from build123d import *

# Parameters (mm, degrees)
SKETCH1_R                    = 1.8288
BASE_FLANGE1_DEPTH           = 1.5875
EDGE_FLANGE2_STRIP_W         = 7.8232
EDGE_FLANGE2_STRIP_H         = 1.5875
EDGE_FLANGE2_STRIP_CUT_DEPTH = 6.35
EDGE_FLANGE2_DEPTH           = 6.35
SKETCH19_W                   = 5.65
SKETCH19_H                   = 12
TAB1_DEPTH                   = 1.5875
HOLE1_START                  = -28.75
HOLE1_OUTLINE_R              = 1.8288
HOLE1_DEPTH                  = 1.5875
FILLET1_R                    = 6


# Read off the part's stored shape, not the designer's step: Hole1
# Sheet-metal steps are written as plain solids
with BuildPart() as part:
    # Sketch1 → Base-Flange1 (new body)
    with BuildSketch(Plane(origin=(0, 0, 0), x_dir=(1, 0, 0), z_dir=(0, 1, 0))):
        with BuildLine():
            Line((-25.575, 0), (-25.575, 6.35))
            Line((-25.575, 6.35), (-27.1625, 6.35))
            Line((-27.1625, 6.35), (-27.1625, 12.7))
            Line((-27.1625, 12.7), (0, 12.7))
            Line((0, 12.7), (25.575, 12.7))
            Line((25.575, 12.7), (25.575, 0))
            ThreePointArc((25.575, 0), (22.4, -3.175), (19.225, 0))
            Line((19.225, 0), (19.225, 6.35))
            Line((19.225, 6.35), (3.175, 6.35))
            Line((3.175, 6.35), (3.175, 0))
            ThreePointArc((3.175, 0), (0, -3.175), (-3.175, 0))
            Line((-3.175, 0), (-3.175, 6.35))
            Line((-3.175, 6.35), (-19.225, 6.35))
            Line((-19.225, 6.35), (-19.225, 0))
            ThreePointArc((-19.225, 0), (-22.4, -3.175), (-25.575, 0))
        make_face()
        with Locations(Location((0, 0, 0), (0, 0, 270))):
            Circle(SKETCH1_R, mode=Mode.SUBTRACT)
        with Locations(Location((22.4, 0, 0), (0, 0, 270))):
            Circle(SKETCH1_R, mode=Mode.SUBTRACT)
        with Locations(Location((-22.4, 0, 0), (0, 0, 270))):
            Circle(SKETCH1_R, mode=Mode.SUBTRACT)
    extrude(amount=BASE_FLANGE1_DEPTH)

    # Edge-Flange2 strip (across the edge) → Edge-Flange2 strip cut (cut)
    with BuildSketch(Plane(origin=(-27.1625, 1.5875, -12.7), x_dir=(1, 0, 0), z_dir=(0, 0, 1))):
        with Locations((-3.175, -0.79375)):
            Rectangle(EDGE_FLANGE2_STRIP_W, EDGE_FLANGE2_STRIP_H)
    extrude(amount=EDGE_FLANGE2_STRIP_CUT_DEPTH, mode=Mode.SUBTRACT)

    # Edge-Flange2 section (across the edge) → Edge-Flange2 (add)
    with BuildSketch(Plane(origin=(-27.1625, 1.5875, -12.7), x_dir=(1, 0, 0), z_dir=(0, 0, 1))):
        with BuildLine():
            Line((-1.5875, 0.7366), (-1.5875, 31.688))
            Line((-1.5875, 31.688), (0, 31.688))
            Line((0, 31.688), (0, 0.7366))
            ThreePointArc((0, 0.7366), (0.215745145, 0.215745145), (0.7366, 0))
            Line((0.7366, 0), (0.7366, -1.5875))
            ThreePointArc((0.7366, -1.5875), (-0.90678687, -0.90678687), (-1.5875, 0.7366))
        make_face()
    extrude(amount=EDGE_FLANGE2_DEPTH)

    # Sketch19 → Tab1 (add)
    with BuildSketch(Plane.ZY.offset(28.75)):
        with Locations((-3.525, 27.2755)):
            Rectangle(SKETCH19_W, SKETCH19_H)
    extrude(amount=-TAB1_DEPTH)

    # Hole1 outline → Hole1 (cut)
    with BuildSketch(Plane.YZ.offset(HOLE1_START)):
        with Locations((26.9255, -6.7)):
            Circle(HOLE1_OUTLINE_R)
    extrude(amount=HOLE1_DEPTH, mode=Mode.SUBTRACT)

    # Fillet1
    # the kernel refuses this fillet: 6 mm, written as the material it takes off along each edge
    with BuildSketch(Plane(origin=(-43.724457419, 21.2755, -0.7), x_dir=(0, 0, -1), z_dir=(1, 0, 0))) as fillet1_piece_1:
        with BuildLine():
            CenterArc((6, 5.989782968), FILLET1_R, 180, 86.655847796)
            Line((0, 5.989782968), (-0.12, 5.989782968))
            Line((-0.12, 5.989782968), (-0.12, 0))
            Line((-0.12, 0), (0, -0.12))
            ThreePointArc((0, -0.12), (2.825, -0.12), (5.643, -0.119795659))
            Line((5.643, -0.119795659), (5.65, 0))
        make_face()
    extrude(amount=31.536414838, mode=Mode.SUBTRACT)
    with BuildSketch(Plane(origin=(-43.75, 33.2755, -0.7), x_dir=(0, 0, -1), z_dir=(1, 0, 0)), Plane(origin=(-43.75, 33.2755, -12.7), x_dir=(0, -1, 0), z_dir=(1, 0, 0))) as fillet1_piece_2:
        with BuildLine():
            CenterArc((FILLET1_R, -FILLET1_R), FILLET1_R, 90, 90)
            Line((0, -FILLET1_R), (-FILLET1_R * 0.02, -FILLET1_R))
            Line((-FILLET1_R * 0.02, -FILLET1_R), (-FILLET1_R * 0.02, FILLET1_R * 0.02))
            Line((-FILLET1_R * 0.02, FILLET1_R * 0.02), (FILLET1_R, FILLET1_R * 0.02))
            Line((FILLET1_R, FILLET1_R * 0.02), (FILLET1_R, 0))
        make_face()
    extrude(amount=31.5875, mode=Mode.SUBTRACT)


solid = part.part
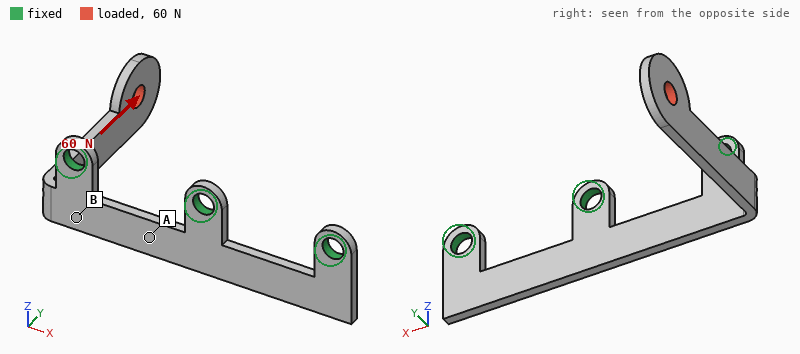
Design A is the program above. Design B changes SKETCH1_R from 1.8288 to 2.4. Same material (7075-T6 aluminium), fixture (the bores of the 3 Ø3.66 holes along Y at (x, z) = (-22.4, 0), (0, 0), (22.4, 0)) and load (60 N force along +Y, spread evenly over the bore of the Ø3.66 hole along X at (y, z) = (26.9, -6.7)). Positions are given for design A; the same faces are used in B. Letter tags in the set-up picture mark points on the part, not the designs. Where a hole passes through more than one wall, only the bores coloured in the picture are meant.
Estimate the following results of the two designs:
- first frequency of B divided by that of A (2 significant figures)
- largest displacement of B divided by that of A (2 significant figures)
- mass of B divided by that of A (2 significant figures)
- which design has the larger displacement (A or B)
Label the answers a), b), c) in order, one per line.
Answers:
a) 1.0
b) 0.91
c) 0.97
d) A
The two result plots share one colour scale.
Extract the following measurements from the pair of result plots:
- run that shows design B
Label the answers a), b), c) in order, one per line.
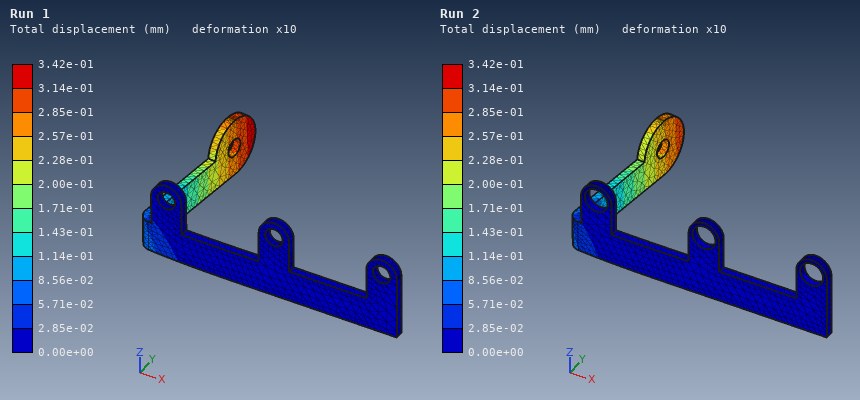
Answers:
a) Run 2
